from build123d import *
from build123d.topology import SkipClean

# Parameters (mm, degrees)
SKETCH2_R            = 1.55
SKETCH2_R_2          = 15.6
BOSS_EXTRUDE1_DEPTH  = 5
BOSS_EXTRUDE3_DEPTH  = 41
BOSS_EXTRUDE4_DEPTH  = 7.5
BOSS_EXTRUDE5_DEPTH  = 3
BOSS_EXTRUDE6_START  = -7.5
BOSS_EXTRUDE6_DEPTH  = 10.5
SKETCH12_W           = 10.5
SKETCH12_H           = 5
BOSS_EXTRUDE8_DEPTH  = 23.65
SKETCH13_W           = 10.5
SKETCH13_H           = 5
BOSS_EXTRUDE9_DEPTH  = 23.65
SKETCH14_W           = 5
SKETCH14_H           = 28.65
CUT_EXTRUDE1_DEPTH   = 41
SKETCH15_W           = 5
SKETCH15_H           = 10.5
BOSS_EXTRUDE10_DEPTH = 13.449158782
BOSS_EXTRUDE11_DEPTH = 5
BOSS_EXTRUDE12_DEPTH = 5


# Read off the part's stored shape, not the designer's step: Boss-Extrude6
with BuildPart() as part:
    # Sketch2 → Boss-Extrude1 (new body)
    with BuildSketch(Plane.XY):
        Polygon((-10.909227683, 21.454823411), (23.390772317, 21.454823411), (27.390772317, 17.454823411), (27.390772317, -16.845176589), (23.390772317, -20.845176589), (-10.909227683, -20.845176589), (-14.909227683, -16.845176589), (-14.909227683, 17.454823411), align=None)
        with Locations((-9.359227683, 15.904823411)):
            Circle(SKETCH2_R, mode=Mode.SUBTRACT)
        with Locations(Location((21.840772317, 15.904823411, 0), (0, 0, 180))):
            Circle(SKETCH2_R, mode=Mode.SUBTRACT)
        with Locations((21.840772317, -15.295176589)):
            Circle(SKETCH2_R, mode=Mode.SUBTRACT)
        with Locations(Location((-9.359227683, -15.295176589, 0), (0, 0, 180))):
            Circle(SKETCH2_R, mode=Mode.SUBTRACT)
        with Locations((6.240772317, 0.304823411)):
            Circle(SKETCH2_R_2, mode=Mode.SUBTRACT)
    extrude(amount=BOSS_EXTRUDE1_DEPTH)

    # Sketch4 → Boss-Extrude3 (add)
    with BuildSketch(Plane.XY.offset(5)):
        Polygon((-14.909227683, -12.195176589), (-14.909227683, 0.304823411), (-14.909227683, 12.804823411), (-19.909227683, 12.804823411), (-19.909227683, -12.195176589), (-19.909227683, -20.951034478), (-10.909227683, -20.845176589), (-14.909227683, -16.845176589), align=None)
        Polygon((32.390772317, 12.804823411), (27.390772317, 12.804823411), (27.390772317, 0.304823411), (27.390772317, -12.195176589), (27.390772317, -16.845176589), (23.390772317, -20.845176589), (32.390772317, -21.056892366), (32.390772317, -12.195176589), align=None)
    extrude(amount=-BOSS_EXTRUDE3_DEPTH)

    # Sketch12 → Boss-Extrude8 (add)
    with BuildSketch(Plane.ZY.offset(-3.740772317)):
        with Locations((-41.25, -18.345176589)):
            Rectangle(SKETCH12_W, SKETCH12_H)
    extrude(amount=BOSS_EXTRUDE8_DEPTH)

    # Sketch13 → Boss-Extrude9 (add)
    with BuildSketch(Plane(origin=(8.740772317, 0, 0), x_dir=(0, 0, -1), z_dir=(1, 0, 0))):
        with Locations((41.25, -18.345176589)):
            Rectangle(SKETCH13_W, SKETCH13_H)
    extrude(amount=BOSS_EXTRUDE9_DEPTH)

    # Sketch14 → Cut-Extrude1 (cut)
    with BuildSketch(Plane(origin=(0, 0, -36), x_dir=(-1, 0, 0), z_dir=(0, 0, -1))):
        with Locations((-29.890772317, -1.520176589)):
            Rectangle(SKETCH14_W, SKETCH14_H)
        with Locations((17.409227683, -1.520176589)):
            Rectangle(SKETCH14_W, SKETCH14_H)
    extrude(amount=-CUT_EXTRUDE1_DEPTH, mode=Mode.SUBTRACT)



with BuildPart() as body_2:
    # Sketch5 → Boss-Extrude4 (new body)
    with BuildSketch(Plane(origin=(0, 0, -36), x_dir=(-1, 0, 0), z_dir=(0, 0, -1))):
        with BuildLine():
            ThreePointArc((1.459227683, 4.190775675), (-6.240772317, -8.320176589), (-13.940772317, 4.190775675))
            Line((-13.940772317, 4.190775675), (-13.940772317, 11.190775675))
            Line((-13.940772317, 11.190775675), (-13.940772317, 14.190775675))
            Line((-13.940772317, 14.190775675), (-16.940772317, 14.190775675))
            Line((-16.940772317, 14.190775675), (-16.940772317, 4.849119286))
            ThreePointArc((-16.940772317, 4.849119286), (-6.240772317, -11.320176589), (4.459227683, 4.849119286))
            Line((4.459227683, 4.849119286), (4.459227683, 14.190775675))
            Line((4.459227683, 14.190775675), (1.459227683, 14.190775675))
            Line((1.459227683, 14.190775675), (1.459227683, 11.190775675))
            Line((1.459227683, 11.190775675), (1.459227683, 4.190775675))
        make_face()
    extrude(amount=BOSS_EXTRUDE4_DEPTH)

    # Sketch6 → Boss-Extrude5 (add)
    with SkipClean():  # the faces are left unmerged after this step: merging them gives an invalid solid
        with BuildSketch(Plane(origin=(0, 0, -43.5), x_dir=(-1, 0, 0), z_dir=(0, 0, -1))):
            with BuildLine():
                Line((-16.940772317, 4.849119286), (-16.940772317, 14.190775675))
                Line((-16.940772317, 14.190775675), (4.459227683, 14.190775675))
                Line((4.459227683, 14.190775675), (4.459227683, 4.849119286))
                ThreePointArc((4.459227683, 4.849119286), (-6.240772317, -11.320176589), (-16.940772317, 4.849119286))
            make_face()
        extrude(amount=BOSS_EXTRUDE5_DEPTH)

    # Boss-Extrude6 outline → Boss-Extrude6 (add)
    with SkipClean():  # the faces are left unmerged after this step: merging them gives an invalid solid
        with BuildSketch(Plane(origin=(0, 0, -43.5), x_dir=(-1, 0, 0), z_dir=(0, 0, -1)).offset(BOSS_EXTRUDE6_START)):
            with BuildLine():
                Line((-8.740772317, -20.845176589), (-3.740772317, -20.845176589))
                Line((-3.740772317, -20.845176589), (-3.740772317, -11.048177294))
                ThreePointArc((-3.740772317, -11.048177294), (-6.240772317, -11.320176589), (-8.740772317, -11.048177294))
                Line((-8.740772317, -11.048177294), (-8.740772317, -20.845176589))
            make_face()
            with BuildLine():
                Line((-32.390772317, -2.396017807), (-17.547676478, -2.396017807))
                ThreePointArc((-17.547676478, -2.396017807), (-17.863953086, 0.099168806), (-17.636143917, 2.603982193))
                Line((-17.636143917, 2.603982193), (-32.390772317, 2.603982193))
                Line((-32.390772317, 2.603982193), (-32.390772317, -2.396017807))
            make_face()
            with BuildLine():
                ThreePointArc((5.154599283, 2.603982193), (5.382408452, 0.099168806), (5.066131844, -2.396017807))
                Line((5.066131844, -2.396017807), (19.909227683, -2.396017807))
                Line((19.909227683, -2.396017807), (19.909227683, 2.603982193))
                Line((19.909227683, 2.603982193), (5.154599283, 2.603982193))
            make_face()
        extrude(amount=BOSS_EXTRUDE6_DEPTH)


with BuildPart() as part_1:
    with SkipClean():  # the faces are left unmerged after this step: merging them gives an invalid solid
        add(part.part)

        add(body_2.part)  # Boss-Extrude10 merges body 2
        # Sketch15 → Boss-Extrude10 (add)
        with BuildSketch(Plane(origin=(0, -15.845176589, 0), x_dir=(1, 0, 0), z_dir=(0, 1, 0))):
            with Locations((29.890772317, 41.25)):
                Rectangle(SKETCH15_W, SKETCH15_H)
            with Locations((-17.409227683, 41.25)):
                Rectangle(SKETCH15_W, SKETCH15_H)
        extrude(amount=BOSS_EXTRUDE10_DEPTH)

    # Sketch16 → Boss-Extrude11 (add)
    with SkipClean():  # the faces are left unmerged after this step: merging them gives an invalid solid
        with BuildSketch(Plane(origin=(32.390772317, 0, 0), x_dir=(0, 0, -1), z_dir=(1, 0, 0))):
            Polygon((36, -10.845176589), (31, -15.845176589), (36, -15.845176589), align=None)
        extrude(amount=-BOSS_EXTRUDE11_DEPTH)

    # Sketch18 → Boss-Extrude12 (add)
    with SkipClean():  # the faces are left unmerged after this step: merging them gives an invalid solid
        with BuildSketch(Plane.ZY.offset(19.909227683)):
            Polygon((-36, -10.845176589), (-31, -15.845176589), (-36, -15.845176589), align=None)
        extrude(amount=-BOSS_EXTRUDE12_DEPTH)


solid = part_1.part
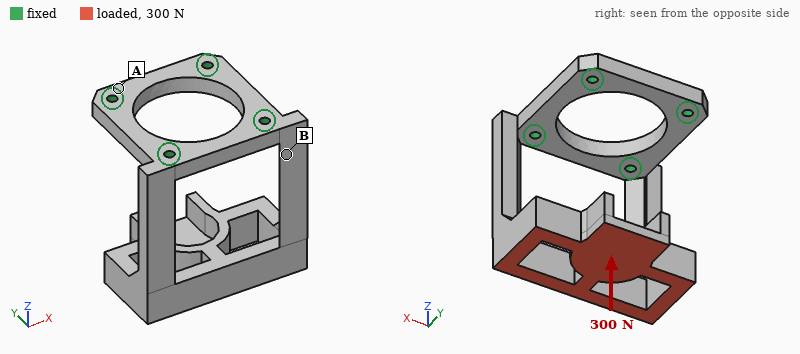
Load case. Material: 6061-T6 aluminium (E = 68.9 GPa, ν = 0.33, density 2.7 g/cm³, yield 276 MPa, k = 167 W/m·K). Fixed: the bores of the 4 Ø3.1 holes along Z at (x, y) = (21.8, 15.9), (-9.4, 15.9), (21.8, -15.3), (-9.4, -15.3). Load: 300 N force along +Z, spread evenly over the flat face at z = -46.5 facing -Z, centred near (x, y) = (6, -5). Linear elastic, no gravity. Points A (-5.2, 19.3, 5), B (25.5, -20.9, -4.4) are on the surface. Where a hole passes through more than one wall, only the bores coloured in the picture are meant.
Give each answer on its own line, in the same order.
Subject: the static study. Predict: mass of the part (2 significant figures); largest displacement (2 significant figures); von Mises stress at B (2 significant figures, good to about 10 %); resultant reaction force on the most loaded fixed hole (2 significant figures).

45 g
0.87 mm
55 MPa
150 N
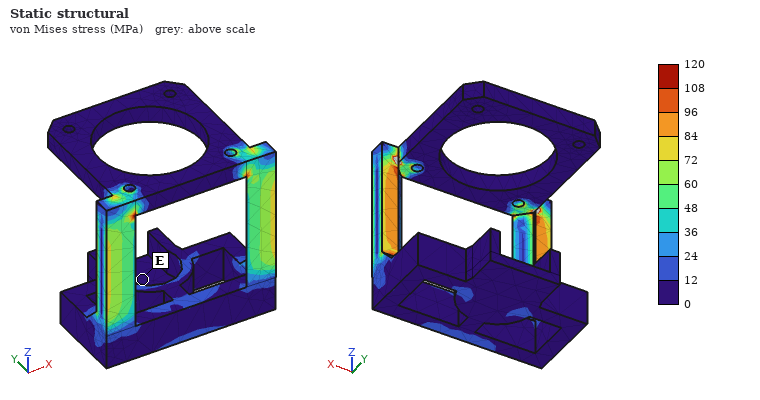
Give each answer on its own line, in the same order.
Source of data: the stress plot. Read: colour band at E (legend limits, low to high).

0 to 12 MPa
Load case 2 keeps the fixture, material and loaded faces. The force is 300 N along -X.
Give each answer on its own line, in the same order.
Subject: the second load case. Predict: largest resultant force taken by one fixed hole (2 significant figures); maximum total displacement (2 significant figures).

290 N
0.46 mm
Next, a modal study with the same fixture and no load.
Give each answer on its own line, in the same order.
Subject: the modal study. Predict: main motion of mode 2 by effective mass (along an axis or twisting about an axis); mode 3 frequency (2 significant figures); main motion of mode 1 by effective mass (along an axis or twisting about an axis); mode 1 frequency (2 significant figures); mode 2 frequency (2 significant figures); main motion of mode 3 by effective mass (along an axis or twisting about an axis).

along X
1800 Hz
along Y
460 Hz
920 Hz
along X
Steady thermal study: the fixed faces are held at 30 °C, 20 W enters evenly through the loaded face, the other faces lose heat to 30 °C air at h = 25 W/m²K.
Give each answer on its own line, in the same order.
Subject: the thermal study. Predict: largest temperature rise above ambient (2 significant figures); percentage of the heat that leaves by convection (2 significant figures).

62 K
38 %
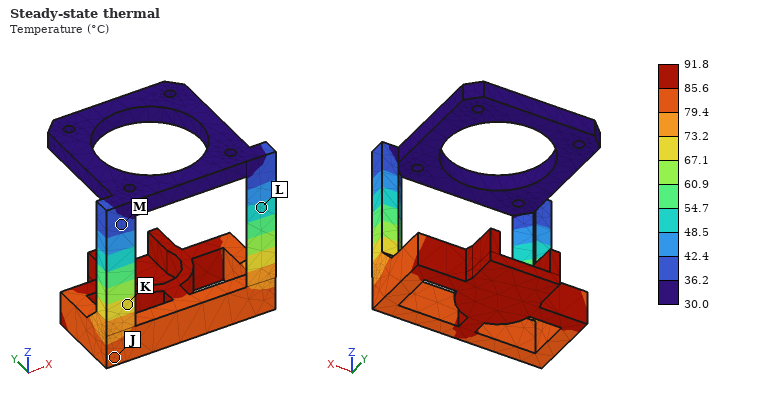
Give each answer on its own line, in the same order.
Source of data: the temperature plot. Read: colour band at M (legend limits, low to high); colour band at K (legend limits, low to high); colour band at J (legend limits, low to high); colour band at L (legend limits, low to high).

36.2 to 42.4 °C
67.1 to 73.2 °C
79.4 to 85.6 °C
48.5 to 54.7 °C
